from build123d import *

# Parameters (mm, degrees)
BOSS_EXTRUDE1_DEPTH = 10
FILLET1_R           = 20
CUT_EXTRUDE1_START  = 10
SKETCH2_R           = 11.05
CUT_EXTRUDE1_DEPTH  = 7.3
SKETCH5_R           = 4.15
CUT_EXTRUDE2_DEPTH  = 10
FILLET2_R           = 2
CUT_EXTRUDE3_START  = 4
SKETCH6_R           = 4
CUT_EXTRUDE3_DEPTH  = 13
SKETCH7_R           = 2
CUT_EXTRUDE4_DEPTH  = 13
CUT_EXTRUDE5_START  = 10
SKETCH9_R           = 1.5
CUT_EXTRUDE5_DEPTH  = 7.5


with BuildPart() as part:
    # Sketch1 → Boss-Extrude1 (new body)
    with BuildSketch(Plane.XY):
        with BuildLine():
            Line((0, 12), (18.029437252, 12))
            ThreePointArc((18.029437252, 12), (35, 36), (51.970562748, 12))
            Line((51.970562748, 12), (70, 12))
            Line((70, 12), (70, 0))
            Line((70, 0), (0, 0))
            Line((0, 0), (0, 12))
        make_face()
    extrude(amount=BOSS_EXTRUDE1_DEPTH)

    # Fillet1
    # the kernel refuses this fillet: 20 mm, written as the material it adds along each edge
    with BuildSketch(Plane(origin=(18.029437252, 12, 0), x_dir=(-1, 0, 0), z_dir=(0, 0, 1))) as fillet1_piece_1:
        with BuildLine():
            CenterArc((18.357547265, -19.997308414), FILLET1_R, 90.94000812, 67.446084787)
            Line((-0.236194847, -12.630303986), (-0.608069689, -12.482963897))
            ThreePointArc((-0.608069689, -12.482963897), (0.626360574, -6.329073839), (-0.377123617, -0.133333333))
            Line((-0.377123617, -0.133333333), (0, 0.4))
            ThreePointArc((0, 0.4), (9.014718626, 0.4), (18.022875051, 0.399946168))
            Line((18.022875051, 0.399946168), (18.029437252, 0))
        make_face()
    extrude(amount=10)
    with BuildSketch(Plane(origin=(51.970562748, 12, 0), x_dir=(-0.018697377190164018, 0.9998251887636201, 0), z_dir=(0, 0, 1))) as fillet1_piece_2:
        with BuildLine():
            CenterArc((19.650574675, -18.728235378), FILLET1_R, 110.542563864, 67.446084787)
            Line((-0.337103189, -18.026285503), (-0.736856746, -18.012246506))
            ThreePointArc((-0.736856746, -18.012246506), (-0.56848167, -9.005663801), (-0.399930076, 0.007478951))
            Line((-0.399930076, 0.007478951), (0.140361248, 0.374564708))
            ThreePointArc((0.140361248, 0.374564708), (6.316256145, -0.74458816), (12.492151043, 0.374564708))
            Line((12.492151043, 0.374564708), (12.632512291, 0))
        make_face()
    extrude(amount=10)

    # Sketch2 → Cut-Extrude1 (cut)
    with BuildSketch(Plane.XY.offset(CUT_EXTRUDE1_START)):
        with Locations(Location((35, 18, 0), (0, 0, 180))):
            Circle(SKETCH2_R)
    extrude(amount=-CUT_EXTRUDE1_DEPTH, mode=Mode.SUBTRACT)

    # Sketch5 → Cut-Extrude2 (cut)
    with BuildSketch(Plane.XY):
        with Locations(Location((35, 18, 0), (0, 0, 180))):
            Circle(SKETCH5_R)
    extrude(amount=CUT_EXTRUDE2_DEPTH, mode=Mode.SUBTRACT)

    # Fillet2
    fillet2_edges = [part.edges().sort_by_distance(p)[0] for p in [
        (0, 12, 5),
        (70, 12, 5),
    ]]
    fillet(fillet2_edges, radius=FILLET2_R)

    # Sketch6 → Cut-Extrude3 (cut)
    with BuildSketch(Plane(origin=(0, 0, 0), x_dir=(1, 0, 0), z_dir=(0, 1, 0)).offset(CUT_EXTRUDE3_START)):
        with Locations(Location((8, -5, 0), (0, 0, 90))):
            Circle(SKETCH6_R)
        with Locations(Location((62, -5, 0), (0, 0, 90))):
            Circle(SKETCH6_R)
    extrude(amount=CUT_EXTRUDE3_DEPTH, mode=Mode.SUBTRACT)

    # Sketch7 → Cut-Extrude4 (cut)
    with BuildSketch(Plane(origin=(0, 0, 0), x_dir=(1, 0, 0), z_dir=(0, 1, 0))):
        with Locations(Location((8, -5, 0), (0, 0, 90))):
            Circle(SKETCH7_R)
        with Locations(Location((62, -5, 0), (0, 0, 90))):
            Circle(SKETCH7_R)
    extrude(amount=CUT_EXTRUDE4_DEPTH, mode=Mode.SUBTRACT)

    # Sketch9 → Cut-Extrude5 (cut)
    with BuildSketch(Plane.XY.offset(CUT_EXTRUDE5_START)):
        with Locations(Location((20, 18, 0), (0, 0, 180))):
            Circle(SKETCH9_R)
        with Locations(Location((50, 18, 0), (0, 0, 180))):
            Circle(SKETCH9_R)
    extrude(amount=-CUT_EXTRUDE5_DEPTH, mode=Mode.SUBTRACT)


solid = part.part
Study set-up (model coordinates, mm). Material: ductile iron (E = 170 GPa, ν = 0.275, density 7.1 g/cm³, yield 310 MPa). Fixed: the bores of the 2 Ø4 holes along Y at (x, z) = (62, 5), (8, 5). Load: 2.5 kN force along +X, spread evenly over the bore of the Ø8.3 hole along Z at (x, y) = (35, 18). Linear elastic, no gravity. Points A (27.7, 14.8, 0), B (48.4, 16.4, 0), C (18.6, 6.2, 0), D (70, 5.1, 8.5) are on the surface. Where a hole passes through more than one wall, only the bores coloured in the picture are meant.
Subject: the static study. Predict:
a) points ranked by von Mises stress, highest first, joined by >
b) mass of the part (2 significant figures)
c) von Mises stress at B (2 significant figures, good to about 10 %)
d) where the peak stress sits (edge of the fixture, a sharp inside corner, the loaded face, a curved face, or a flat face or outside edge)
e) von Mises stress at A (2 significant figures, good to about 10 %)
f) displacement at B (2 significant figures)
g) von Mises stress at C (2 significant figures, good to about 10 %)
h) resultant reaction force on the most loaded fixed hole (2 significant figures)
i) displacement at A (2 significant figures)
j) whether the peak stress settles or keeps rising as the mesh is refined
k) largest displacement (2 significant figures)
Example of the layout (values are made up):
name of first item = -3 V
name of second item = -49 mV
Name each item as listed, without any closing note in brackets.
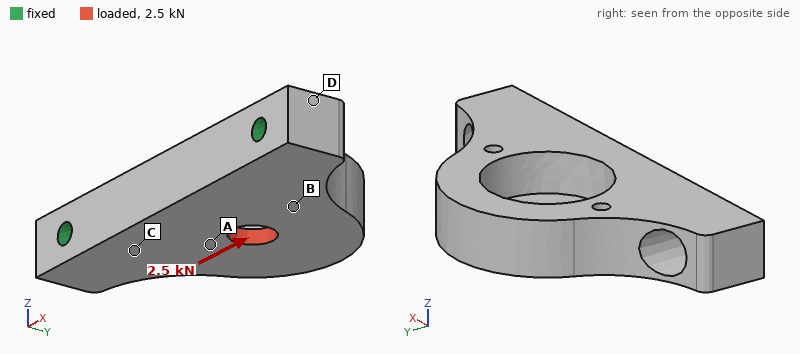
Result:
points ranked by von Mises stress, highest first, joined by > = A > B > C > D
mass of the part = 89 g
von Mises stress at B = 26 MPa
where the peak stress sits = edge of the fixture
von Mises stress at A = 34 MPa
displacement at B = 3.8 µm
von Mises stress at C = 18 MPa
resultant reaction force on the most loaded fixed hole = 1.5 kN
displacement at A = 3.9 µm
whether the peak stress settles or keeps rising as the mesh is refined = keeps rising
largest displacement = 6.6 µm
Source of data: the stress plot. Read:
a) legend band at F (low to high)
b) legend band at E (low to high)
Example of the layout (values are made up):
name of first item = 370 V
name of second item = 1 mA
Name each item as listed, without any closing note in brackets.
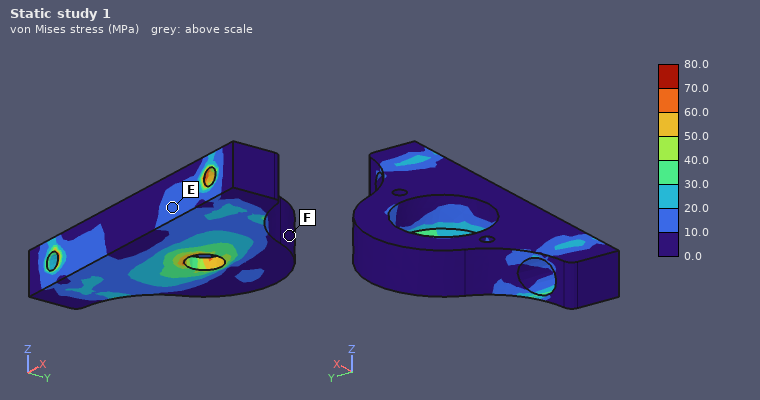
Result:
legend band at F = 0.0 to 10.0 MPa
legend band at E = 10.0 to 20.0 MPa
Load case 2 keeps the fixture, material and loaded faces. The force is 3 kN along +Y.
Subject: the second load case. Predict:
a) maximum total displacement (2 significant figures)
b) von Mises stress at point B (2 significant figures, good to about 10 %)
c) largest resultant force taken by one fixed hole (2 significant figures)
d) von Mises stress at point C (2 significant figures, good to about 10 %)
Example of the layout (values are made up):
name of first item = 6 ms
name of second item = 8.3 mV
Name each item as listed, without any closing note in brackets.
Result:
maximum total displacement = 42 µm
von Mises stress at point B = 21 MPa
largest resultant force taken by one fixed hole = 1.8 kN
von Mises stress at point C = 28 MPa
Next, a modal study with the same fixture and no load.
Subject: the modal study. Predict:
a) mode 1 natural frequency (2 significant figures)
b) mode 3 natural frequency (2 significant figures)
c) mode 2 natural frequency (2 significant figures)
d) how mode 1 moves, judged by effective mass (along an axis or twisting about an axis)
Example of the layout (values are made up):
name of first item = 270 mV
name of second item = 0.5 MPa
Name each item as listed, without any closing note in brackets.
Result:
mode 1 natural frequency = 3600 Hz
mode 3 natural frequency = 12 kHz
mode 2 natural frequency = 12 kHz
how mode 1 moves, judged by effective mass = along Z
